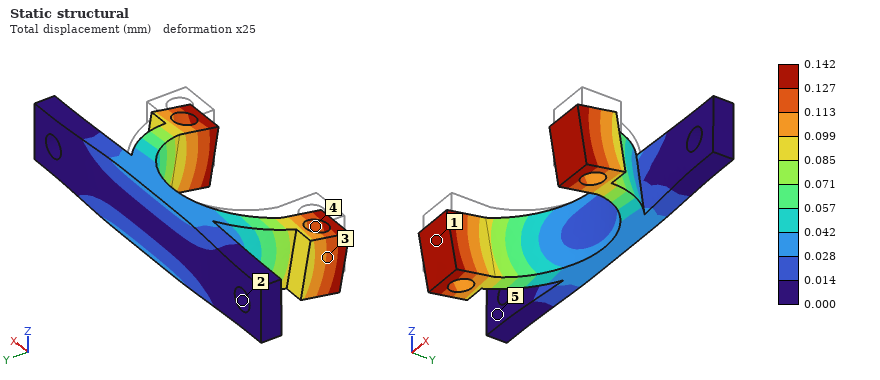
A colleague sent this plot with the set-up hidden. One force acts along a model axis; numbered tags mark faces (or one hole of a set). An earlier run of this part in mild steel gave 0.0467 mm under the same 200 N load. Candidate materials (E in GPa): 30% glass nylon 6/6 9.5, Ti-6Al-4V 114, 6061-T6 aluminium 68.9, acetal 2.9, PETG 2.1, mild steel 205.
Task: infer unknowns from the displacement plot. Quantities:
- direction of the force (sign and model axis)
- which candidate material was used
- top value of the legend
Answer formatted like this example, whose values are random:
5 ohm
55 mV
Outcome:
-Z
6061-T6 aluminium
0.142 mm
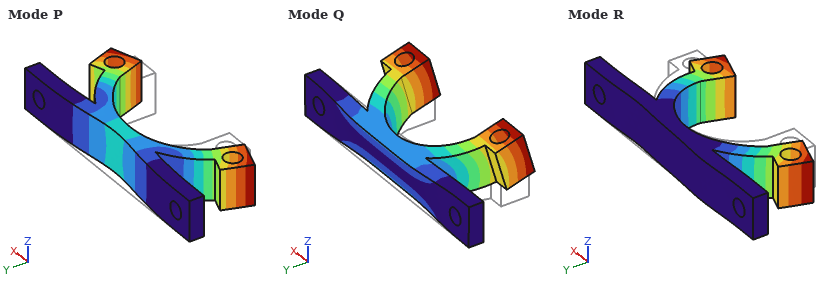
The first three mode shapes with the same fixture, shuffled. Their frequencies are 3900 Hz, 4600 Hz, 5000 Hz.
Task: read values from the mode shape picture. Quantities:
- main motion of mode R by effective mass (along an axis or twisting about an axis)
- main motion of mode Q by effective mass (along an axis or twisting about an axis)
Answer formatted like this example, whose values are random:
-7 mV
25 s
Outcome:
along X
along Z
